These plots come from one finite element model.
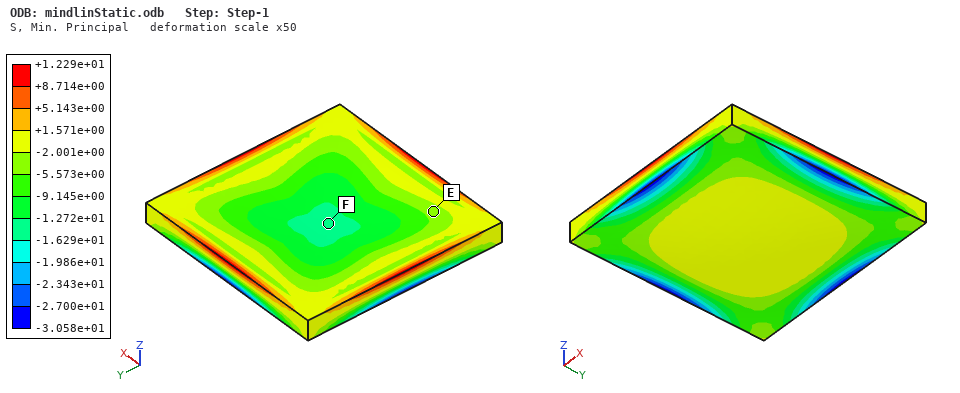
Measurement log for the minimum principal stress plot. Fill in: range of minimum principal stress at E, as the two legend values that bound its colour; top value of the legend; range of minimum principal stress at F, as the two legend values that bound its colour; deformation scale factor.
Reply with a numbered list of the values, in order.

1. -5.573e+00 to -2.001e+00
2. +1.229e+01
3. -1.629e+01 to -1.272e+01
4. 50
